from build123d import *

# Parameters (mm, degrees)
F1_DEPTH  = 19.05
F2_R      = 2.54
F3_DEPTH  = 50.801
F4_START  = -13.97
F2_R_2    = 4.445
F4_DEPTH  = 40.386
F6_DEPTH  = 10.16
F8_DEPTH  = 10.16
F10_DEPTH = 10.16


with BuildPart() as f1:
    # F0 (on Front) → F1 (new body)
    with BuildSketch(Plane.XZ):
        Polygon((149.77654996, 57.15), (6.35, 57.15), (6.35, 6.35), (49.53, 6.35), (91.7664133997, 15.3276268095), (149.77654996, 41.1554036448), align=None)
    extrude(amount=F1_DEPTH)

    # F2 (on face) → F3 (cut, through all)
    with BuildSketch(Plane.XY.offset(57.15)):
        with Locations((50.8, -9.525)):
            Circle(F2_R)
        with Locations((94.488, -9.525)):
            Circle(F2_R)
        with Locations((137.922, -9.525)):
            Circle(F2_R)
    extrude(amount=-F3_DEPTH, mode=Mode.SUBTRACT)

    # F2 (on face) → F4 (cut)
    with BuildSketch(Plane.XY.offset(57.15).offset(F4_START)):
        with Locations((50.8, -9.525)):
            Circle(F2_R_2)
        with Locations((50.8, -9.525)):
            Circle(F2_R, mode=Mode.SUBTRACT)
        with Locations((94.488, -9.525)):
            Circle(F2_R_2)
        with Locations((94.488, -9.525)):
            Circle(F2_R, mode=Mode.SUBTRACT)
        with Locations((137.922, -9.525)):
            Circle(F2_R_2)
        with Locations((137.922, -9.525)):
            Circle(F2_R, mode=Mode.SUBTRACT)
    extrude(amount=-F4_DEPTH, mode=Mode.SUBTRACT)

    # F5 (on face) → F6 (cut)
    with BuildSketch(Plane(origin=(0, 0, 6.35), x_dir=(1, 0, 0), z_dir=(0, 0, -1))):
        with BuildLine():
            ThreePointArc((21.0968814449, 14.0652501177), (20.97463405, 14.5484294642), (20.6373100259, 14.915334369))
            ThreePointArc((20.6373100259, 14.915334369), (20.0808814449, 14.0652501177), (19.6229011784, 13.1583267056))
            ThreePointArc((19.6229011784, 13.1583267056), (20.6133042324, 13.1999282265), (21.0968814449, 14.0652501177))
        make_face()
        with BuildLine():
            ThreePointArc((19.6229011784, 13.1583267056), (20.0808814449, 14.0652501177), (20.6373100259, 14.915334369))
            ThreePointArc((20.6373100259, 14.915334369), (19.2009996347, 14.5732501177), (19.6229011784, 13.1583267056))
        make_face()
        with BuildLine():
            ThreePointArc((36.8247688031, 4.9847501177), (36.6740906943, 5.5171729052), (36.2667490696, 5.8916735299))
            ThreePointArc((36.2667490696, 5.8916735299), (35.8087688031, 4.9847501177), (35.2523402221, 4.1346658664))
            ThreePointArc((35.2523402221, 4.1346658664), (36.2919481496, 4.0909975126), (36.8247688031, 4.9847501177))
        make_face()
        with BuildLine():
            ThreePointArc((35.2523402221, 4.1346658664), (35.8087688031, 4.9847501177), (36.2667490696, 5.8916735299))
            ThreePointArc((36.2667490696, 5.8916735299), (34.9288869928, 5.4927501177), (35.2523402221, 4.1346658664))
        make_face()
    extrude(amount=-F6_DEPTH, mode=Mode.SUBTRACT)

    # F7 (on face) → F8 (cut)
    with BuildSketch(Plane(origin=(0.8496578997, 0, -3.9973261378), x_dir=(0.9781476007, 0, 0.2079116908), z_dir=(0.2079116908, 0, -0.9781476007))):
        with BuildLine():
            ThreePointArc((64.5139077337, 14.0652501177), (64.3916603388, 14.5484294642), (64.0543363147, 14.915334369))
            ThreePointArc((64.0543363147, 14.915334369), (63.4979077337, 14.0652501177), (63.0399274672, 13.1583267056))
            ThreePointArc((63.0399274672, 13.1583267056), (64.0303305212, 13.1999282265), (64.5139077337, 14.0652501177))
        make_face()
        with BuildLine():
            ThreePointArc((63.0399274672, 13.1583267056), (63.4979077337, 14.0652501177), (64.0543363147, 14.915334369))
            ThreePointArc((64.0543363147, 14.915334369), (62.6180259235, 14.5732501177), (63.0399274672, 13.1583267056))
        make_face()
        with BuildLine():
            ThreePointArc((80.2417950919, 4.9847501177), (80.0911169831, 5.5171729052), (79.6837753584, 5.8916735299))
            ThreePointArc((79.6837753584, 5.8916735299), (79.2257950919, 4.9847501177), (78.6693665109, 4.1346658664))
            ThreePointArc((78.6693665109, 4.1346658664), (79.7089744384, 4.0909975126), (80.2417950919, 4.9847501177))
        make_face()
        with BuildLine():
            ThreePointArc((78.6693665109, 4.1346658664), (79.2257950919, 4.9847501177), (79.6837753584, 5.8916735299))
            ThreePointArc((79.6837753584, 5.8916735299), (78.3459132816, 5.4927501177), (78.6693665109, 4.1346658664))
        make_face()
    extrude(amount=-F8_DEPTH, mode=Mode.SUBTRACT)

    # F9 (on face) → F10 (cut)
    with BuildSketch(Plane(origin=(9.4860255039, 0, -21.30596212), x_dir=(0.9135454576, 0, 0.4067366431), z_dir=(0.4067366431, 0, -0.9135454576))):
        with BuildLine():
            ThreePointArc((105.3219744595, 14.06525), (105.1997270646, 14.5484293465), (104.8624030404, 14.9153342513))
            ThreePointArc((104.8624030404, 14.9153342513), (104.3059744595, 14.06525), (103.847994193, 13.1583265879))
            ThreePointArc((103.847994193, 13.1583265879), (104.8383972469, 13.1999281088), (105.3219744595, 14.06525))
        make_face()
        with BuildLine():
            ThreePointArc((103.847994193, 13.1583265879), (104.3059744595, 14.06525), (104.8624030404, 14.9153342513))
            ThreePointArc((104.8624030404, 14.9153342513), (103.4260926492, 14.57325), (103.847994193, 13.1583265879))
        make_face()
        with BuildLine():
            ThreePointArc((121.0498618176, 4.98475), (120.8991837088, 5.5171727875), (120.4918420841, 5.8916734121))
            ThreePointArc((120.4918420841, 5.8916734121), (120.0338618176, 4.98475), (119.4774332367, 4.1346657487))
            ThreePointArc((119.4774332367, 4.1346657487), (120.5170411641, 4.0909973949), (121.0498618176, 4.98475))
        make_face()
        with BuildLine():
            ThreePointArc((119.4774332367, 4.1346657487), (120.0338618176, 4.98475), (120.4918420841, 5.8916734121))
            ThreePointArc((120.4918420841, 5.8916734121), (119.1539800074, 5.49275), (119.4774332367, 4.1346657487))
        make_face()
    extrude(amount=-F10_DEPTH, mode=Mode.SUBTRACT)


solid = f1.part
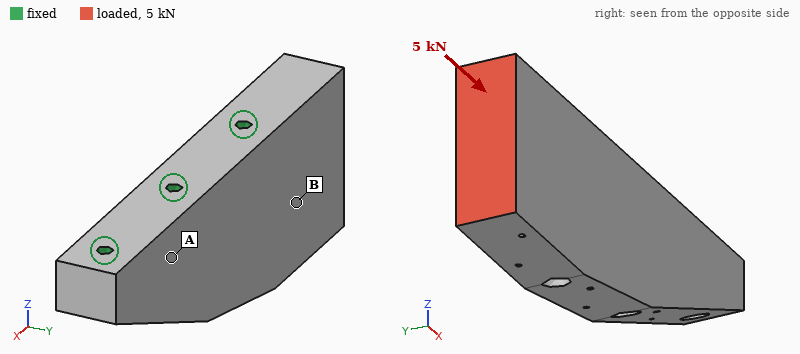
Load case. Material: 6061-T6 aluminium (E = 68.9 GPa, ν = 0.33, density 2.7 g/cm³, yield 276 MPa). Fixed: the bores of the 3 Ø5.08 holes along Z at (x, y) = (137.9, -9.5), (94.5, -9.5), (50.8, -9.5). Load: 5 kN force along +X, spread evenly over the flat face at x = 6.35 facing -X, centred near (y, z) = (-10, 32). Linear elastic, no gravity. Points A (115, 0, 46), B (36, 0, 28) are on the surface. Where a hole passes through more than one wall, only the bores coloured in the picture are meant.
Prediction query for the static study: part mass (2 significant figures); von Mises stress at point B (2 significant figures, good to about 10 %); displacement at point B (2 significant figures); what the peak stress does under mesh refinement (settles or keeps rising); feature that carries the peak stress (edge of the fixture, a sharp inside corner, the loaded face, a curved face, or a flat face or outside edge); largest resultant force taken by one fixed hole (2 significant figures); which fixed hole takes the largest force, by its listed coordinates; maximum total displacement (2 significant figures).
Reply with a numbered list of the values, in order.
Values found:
1. 290 g
2. 5.5 MPa
3. 7.2 µm
4. keeps rising
5. edge of the fixture
6. 3.2 kN
7. (50.8, -9.5)
8. 16 µm
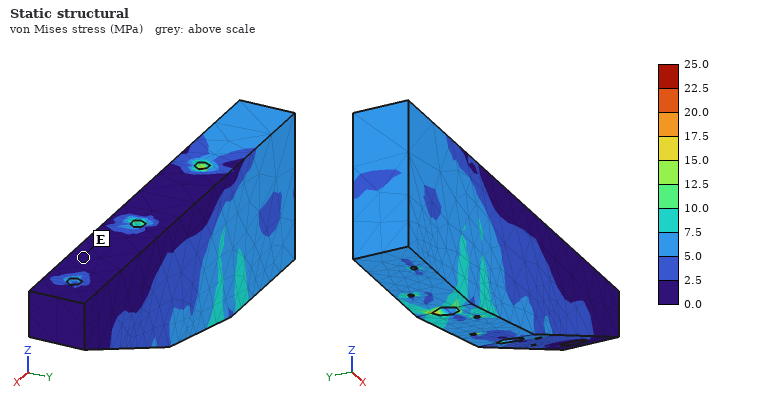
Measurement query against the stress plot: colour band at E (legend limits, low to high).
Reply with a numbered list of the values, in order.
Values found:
1. 0.0 to 2.5 MPa
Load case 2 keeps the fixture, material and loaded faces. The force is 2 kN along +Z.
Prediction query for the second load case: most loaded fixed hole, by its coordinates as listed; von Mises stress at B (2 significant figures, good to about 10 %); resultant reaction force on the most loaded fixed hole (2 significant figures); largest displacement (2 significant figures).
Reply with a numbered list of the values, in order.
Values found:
1. (50.8, -9.5)
2. 5.4 MPa
3. 3.5 kN
4. 24 µm
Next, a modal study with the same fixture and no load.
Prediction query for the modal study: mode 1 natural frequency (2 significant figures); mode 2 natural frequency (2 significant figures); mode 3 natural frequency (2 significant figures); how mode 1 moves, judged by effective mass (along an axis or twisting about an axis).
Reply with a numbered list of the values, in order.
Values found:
1. 3500 Hz
2. 5900 Hz
3. 6800 Hz
4. along Y
